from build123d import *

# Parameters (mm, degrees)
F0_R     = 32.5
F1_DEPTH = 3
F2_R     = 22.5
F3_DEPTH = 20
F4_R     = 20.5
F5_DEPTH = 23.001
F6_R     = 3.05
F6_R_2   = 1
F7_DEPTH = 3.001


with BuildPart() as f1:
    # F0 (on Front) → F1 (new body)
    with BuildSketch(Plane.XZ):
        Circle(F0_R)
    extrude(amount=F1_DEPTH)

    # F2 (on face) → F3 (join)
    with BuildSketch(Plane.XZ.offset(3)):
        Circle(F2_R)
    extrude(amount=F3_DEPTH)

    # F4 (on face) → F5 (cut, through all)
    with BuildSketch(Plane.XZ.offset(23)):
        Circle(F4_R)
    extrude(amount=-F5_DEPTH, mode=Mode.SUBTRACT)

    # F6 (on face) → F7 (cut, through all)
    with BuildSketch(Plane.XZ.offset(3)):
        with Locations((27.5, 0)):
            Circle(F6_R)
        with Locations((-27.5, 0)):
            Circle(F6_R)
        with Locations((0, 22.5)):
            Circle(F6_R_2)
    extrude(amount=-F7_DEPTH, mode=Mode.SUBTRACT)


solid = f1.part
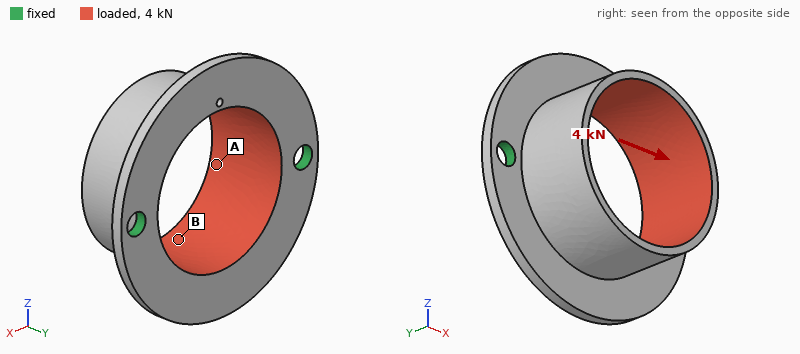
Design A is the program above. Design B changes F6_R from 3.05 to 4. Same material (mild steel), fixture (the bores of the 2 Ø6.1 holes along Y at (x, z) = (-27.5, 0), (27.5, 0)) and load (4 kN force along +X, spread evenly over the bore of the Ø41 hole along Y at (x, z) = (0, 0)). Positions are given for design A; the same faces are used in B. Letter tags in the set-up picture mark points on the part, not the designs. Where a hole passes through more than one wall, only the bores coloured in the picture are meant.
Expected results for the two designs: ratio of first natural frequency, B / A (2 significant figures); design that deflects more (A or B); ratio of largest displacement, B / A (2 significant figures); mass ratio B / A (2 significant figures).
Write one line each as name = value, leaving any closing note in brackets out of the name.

ratio of first natural frequency, B / A = 1.2
design that deflects more = A
ratio of largest displacement, B / A = 0.90
mass ratio B / A = 0.99
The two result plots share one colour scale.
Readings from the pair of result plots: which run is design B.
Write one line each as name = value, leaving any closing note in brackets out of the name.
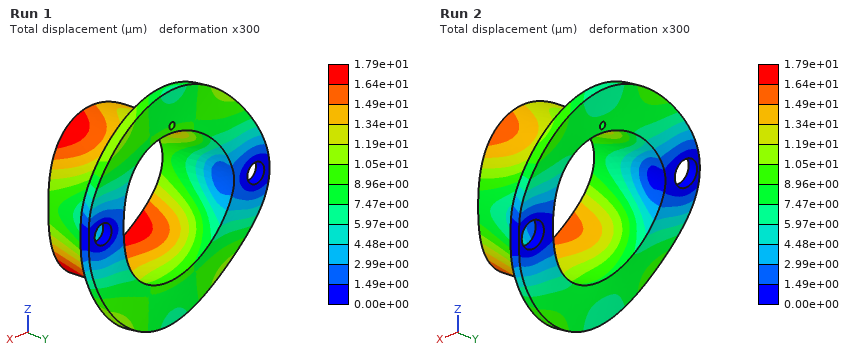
which run is design B = Run 2
